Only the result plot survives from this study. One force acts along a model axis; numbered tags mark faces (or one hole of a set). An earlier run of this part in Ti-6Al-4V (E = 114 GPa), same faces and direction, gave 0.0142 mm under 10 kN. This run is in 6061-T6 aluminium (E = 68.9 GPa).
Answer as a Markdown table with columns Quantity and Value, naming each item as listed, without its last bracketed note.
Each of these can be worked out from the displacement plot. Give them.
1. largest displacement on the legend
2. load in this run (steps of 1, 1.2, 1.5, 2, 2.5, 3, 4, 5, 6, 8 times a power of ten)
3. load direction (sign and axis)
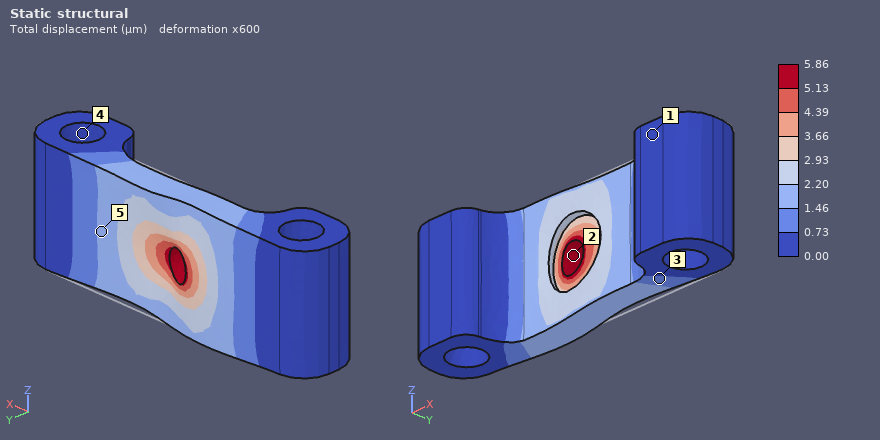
| Quantity | Value |
|---|---|
| largest displacement on the legend | 5.86 µm |
| load in this run | 2.5 kN |
| load direction | -X |
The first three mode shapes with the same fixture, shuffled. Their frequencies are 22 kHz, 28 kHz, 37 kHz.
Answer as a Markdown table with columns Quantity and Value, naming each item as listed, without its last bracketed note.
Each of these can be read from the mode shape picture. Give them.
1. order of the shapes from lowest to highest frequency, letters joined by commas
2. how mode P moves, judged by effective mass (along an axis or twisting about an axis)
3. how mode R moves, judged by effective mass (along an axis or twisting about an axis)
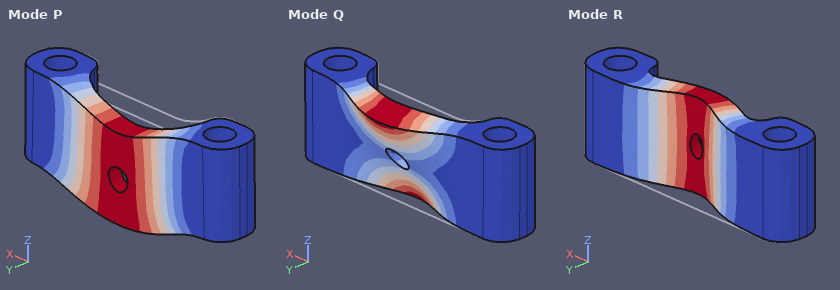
| Quantity | Value |
|---|---|
| order of the shapes from lowest to highest frequency, letters joined by commas | R, Q, P |
| how mode P moves, judged by effective mass | along Z |
| how mode R moves, judged by effective mass | along Y |
